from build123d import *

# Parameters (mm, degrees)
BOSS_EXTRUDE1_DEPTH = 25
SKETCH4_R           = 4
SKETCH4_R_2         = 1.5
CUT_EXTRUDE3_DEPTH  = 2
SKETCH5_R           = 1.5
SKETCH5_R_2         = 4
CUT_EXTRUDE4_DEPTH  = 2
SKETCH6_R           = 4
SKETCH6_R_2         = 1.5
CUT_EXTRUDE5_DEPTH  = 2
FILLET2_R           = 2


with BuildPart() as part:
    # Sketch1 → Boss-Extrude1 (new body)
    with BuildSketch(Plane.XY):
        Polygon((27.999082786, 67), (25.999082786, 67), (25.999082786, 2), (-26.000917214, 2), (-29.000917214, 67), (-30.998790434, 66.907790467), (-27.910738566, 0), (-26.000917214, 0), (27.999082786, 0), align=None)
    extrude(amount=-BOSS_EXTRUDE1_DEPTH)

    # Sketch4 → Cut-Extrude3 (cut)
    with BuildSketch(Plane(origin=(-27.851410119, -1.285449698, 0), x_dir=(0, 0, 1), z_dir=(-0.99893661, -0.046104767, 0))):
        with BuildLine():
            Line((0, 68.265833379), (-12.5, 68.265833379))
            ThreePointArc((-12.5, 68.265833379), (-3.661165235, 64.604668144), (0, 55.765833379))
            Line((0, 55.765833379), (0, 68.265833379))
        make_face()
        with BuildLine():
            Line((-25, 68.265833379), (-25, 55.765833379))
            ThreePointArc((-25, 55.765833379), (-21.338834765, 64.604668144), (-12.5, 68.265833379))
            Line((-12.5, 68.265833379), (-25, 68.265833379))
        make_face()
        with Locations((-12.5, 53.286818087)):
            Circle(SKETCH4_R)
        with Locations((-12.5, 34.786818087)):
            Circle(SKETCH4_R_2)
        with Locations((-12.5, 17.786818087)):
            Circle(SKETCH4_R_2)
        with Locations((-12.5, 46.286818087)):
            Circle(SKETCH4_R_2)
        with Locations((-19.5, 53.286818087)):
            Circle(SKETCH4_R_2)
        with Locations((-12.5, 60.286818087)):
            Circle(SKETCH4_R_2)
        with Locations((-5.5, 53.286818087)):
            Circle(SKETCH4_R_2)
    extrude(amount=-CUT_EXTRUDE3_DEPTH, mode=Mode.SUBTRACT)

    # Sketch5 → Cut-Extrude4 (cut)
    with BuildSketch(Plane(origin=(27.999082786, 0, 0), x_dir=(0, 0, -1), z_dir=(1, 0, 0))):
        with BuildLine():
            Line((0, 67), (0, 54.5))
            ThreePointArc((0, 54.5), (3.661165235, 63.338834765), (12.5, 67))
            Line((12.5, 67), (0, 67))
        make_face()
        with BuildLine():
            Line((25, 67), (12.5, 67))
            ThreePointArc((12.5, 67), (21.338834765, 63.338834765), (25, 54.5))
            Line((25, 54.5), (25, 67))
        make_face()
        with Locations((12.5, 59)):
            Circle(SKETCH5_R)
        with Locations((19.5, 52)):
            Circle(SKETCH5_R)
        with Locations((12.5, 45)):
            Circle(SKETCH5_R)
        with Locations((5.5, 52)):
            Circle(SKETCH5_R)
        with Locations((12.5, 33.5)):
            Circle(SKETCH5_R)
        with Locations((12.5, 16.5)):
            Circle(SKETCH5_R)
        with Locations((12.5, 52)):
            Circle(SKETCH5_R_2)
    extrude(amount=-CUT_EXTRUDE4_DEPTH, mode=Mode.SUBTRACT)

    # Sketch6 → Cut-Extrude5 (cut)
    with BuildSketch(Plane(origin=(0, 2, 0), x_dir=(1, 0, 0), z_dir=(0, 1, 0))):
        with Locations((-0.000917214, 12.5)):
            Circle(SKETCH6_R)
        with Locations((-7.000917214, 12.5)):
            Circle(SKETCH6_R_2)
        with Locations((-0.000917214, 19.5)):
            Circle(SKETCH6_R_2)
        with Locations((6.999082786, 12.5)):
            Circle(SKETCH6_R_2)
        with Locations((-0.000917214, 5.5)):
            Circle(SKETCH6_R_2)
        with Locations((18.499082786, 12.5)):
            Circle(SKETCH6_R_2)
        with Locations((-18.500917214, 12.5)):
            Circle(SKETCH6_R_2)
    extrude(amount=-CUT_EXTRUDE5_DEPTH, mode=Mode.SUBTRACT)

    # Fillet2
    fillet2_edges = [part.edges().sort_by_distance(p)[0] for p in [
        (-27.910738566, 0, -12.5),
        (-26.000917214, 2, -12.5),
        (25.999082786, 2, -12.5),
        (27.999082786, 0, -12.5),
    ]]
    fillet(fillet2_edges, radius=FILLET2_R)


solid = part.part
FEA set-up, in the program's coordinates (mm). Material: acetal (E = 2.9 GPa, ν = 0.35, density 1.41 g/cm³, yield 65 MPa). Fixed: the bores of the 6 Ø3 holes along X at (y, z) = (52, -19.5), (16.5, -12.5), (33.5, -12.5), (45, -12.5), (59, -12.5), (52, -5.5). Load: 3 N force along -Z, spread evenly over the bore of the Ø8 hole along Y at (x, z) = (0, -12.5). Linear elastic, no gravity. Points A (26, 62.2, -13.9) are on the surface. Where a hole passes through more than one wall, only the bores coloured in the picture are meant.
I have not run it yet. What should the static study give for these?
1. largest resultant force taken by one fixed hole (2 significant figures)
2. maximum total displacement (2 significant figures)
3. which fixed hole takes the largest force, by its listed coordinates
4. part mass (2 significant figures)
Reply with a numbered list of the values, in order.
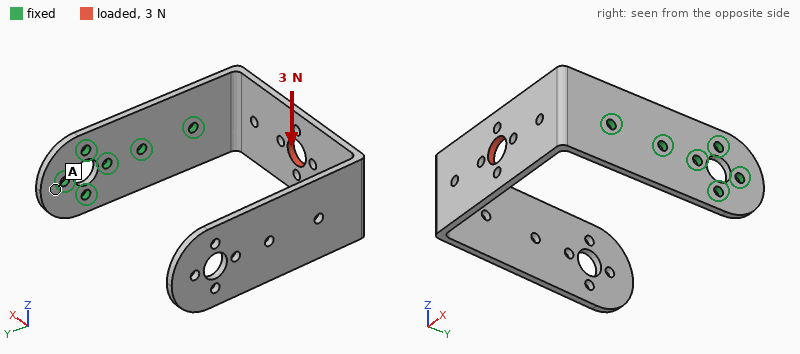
1. 4.6 N
2. 1.1 mm
3. (16.5, -12.5)
4. 12 g
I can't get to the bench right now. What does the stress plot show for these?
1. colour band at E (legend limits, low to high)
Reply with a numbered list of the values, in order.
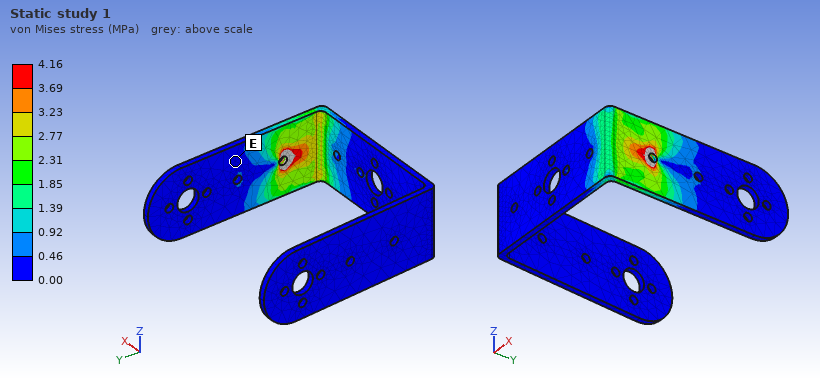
1. 0.00 to 0.46 MPa
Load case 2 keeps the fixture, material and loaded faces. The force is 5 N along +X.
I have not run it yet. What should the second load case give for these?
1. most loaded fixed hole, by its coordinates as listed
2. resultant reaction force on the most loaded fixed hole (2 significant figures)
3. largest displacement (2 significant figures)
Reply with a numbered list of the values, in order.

1. (16.5, -12.5)
2. 6.6 N
3. 1.00 mm
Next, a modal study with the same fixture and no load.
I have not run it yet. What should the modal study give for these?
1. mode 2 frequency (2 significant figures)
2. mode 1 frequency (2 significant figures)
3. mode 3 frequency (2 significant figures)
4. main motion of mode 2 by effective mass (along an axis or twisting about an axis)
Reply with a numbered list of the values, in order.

1. 59 Hz
2. 38 Hz
3. 110 Hz
4. along Z
